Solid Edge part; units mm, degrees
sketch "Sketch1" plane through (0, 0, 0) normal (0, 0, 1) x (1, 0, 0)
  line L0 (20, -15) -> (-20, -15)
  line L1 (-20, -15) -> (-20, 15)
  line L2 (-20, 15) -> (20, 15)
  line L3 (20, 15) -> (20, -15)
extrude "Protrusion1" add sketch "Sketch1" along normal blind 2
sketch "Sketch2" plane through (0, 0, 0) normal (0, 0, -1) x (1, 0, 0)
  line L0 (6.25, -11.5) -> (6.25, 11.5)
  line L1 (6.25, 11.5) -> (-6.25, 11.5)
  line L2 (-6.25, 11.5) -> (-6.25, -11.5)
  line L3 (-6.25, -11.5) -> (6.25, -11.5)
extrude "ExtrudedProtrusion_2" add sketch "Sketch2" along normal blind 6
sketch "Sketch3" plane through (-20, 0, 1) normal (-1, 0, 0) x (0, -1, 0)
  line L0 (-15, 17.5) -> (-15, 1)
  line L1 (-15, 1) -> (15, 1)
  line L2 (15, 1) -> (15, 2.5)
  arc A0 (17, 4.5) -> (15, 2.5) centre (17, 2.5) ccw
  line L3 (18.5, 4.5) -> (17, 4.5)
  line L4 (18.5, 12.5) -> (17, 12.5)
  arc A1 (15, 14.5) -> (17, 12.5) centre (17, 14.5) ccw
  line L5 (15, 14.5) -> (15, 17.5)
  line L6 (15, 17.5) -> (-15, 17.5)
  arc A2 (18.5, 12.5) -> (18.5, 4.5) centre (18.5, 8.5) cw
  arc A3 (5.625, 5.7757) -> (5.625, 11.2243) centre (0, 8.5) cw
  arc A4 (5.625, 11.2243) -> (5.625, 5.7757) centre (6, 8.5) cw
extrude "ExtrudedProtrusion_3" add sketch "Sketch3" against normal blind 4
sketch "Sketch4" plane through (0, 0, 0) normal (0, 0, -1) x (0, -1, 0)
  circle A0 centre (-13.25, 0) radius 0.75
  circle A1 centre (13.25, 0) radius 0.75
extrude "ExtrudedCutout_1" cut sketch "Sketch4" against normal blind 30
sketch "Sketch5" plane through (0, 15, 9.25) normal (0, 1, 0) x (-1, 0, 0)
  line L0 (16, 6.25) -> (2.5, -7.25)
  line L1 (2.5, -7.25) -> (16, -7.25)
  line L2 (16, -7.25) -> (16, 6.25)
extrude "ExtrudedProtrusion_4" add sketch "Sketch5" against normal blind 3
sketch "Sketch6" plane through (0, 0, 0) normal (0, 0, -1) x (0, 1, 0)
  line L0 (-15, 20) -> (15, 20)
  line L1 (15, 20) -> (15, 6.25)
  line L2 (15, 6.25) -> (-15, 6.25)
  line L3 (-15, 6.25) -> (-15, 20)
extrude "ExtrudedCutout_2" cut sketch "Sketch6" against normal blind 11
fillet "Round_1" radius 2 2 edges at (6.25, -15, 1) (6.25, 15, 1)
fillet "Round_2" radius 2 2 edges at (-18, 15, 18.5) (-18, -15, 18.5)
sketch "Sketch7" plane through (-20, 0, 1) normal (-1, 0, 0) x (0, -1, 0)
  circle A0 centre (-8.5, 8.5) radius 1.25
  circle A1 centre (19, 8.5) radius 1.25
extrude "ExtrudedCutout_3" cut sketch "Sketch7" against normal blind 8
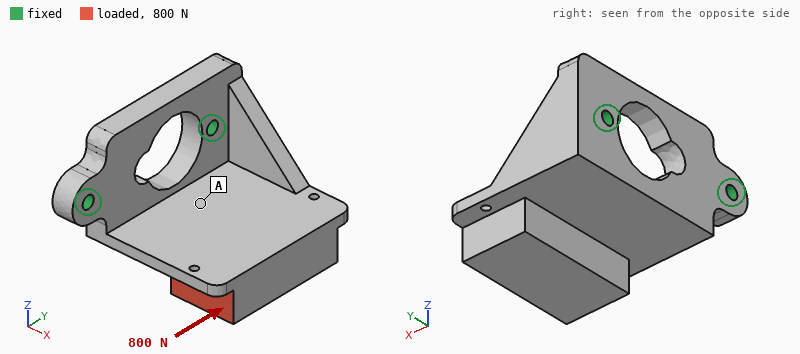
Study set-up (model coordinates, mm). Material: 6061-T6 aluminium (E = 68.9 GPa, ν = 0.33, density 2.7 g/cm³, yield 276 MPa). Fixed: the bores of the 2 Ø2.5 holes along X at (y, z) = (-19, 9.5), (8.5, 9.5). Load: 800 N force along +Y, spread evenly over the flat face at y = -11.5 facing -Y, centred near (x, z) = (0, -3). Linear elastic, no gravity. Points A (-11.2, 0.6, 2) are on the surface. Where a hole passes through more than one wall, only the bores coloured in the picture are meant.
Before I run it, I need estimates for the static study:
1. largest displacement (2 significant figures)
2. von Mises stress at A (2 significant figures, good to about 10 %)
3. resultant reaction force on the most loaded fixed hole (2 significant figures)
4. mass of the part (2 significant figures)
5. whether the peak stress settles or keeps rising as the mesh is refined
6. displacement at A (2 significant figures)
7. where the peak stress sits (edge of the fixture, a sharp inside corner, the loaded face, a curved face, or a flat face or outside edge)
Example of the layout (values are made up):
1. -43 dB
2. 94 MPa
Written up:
1. 0.13 mm
2. 19 MPa
3. 740 N
4. 14 g
5. keeps rising
6. 0.031 mm
7. edge of the fixture
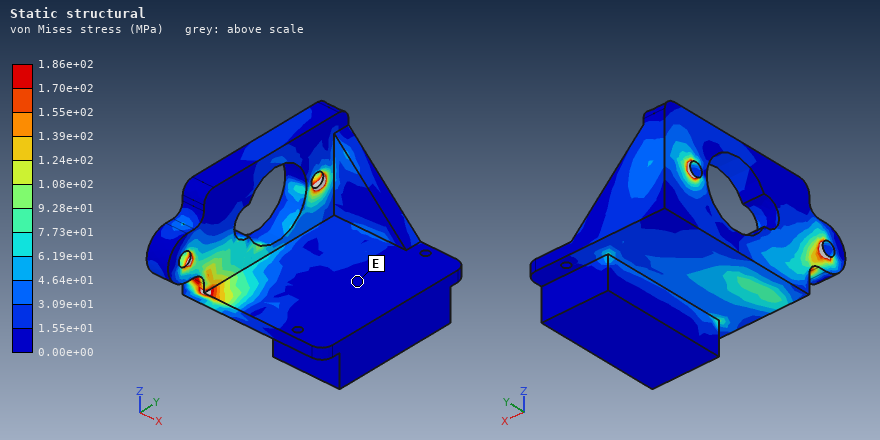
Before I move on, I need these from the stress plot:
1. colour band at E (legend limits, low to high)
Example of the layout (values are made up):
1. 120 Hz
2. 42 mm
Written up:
1. 0.00e+00 to 1.55e+01 MPa
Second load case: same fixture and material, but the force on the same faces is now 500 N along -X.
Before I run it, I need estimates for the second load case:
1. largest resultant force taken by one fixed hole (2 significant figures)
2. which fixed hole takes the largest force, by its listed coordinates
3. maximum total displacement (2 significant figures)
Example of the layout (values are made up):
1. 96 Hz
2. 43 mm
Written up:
1. 370 N
2. (-19, 9.5)
3. 0.24 mm
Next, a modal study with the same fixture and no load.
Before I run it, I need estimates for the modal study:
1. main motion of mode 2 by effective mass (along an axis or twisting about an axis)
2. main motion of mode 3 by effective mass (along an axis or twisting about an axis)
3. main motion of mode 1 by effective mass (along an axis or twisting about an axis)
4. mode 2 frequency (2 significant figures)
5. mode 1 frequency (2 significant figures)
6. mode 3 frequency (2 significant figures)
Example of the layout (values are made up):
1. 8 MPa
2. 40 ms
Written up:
1. along Y
2. along X
3. along Z
4. 5700 Hz
5. 2300 Hz
6. 7800 Hz
